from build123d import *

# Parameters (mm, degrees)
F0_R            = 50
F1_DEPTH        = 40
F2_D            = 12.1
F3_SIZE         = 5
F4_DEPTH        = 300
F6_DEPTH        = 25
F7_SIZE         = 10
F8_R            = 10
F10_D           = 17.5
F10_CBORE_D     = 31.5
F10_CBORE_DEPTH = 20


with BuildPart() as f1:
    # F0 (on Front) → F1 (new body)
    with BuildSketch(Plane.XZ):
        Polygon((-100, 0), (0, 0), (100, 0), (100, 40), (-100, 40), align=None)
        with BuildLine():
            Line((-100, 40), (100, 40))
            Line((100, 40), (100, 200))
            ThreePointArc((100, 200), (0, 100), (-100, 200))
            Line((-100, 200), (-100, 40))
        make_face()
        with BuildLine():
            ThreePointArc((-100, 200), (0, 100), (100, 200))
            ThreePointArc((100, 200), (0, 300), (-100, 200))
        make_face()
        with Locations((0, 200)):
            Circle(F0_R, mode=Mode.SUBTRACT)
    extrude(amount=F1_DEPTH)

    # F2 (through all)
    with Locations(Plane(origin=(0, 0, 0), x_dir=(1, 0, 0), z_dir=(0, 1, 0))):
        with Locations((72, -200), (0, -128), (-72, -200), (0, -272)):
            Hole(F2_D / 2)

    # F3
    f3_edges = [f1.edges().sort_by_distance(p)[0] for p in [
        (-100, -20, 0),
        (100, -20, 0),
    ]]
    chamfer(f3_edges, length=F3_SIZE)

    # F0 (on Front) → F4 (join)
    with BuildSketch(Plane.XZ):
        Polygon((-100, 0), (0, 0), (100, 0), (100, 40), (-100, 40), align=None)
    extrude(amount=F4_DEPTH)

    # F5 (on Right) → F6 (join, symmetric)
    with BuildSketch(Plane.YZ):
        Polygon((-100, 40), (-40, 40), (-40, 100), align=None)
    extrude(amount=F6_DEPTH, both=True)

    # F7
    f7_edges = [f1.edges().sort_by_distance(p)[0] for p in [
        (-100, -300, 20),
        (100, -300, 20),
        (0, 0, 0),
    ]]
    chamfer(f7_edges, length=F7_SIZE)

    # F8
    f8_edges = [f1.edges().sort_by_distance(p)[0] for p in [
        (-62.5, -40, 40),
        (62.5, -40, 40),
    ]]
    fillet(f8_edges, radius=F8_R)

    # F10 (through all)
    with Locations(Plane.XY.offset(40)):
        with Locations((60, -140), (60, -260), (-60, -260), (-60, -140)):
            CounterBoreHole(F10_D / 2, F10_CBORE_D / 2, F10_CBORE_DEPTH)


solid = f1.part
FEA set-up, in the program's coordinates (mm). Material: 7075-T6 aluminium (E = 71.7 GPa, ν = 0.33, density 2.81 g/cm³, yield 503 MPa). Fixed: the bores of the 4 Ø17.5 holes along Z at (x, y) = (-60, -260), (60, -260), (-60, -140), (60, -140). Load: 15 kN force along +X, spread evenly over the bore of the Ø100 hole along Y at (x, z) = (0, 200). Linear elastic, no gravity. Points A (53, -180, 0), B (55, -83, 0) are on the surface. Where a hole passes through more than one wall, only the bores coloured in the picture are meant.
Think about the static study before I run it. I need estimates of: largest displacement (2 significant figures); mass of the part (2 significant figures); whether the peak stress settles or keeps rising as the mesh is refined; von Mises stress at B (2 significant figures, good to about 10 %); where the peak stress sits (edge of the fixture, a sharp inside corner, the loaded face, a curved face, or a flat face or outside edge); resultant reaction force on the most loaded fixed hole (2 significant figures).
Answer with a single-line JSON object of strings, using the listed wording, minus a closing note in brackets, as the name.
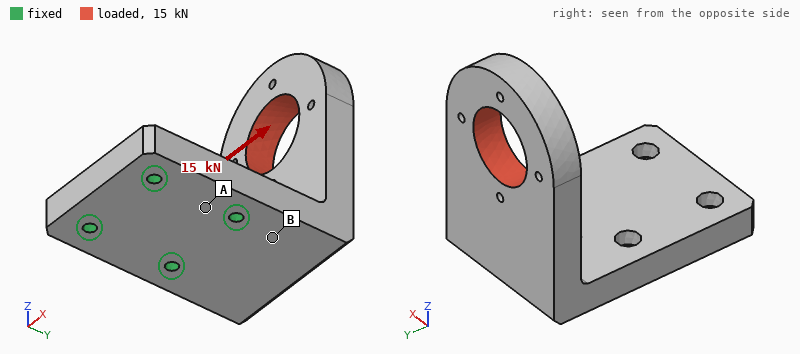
{"largest displacement": "0.49 mm", "mass of the part": "11 kg", "whether the peak stress settles or keeps rising as the mesh is refined": "keeps rising", "von Mises stress at B": "21 MPa", "where the peak stress sits": "edge of the fixture", "resultant reaction force on the most loaded fixed hole": "29 kN"}
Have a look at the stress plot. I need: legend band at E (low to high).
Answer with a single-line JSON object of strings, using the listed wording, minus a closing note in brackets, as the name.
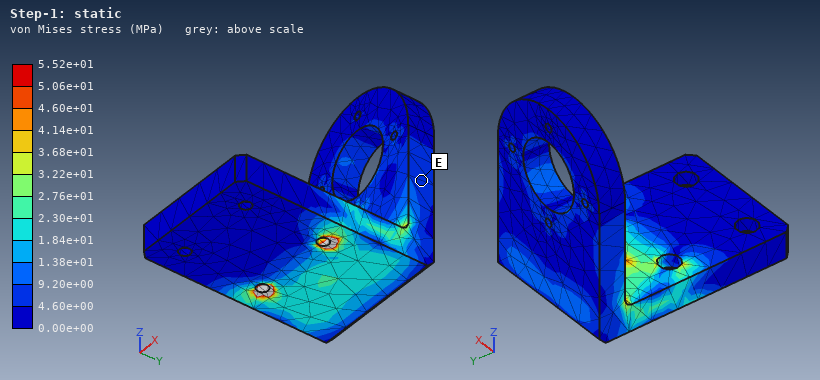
{"legend band at E": "4.60e+00 to 9.20e+00 MPa"}
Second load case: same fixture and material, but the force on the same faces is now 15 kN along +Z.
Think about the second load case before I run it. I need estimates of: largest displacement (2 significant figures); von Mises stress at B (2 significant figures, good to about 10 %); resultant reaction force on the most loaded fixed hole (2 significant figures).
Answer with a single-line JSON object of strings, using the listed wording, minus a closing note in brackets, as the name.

{"largest displacement": "0.57 mm", "von Mises stress at B": "15 MPa", "resultant reaction force on the most loaded fixed hole": "15 kN"}
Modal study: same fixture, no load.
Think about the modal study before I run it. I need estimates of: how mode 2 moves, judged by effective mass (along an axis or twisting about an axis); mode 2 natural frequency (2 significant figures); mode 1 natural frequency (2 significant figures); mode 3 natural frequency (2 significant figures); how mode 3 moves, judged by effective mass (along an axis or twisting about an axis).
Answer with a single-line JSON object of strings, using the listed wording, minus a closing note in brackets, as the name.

{"how mode 2 moves, judged by effective mass": "along X", "mode 2 natural frequency": "570 Hz", "mode 1 natural frequency": "320 Hz", "mode 3 natural frequency": "980 Hz", "how mode 3 moves, judged by effective mass": "along Z"}
